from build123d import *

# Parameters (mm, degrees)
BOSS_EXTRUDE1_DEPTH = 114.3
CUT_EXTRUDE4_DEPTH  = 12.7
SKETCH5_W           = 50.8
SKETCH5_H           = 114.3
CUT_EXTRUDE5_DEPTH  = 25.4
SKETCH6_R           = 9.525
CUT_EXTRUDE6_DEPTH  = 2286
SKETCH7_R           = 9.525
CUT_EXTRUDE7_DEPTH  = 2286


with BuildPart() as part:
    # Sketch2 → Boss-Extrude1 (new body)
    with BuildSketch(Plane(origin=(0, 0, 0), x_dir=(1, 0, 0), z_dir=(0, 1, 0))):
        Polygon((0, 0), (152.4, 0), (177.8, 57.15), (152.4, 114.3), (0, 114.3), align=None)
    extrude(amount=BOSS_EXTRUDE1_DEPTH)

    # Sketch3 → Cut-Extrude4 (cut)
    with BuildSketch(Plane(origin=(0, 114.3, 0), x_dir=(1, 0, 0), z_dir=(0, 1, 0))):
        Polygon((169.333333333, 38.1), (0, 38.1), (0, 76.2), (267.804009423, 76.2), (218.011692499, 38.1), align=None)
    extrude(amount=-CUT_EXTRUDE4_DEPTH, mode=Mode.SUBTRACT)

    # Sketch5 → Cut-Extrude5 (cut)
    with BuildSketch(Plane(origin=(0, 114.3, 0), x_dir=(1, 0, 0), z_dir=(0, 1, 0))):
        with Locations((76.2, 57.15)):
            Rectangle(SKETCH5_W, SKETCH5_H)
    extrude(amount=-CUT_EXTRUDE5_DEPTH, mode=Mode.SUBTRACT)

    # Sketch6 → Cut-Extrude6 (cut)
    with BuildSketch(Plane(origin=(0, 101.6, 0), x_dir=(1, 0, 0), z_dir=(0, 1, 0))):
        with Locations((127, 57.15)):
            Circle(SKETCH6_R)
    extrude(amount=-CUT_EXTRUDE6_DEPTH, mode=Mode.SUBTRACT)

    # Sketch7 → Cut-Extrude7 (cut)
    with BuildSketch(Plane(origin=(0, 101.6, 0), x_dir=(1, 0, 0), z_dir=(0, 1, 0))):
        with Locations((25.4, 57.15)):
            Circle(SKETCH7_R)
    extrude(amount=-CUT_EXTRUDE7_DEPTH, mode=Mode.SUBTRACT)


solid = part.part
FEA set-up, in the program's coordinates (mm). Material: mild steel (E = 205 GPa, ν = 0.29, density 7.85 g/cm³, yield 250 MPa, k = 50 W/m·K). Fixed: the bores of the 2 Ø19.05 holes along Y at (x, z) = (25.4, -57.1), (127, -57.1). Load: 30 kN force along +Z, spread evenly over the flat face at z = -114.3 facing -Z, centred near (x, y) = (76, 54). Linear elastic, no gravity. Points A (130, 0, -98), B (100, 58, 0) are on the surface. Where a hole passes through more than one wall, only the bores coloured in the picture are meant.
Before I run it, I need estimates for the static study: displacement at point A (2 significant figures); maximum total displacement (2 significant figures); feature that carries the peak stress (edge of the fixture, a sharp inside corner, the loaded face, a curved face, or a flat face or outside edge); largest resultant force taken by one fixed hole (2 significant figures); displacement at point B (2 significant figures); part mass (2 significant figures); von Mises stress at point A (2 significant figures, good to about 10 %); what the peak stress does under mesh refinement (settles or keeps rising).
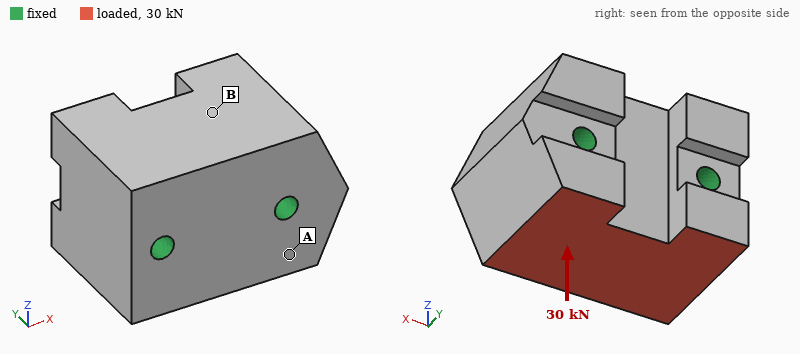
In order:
0.40 µm
1.0 µm
edge of the fixture
15 kN
0.19 µm
15 kg
2.0 MPa
keeps rising
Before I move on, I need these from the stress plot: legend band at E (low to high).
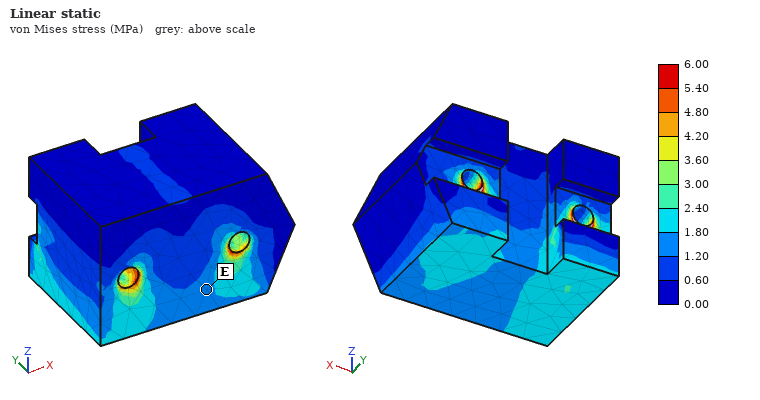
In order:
1.20 to 1.80 MPa
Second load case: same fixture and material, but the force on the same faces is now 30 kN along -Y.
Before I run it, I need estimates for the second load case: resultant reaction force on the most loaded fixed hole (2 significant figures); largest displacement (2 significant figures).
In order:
15 kN
4.0 µm
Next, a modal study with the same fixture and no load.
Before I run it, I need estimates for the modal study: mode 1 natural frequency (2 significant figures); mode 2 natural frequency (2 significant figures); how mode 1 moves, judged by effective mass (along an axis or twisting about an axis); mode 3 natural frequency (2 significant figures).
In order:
9100 Hz
9600 Hz
twisting about X
9900 Hz
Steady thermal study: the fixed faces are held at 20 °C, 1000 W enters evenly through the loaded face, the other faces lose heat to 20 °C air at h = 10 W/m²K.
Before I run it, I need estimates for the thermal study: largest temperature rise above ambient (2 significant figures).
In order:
78 K
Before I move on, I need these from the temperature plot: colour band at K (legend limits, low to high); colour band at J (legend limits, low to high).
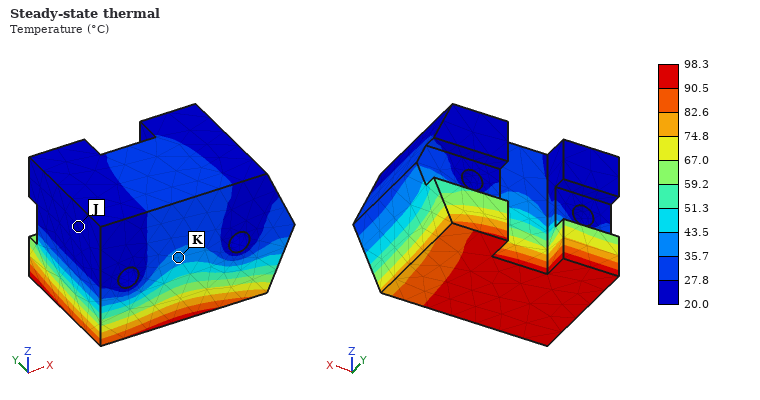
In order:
35.7 to 43.5 °C
20.0 to 27.8 °C
